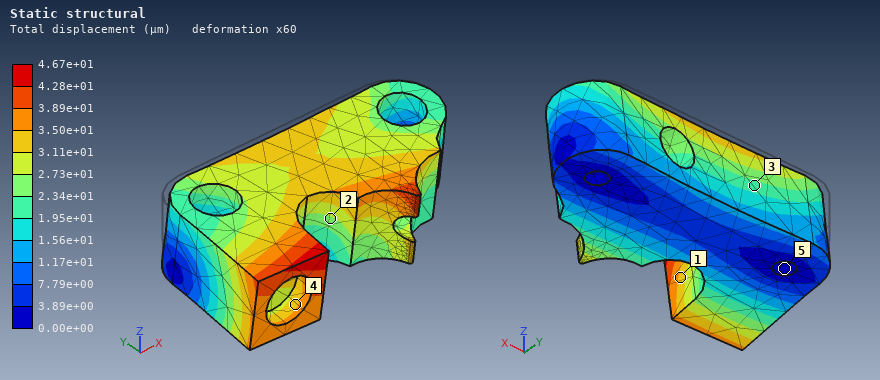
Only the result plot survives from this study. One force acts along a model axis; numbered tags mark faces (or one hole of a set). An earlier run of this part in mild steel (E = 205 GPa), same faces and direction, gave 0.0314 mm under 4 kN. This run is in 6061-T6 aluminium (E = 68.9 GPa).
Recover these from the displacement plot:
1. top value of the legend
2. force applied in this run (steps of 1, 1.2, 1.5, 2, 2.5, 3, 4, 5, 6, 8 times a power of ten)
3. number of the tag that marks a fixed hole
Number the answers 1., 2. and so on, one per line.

1. 4.67e+01 µm
2. 2 kN
3. 5
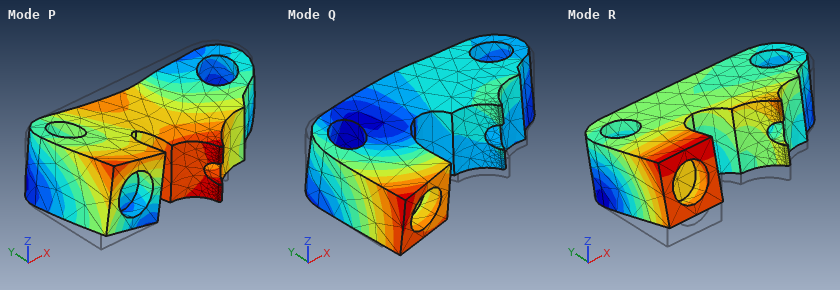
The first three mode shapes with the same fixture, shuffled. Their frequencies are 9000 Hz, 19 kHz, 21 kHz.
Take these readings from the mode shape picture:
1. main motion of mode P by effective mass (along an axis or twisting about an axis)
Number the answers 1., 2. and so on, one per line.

1. along Z
